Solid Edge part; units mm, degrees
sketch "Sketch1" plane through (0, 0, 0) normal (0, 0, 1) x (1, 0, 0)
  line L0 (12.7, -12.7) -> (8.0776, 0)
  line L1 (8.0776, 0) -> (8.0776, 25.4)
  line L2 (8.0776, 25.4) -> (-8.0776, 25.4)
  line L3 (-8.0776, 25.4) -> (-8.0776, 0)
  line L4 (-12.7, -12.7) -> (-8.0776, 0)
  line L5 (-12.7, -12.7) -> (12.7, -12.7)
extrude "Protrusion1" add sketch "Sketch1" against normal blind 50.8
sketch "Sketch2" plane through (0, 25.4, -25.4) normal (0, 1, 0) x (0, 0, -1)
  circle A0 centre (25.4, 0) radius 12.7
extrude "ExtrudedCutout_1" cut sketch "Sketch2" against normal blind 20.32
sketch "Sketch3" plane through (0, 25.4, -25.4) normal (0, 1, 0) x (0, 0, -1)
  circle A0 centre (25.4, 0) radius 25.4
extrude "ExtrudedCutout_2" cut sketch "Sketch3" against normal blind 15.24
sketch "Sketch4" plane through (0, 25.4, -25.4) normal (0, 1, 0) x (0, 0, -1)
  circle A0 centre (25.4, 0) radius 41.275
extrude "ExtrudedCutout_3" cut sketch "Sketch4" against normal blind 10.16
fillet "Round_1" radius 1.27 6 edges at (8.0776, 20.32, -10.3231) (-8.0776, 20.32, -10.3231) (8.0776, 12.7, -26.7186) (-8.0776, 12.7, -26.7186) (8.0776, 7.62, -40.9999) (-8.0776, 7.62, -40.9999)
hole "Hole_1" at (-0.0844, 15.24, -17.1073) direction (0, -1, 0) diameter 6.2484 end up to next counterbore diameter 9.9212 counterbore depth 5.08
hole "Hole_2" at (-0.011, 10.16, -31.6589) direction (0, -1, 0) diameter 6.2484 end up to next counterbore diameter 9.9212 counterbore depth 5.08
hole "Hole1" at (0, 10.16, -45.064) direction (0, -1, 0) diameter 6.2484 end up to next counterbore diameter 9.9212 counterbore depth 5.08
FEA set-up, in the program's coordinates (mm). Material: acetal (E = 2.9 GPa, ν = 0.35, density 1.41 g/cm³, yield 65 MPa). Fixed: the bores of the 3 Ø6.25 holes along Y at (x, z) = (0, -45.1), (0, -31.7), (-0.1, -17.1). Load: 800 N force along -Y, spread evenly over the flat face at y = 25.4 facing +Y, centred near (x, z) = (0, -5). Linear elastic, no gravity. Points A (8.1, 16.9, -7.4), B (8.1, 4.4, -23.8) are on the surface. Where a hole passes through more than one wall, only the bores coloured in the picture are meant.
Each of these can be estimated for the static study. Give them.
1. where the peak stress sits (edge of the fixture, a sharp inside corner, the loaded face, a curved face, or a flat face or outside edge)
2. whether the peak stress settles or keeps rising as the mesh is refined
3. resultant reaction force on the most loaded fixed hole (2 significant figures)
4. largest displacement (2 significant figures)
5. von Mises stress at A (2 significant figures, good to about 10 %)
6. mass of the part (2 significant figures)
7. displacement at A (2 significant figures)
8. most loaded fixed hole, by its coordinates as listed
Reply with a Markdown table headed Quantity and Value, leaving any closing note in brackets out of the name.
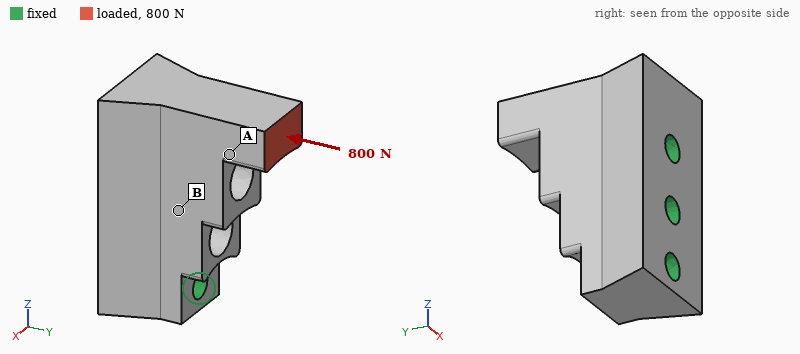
| Quantity | Value |
|---|---|
| where the peak stress sits | edge of the fixture |
| whether the peak stress settles or keeps rising as the mesh is refined | keeps rising |
| resultant reaction force on the most loaded fixed hole | 860 N |
| largest displacement | 0.11 mm |
| von Mises stress at A | 4.4 MPa |
| mass of the part | 31 g |
| displacement at A | 0.054 mm |
| most loaded fixed hole, by its coordinates as listed | (-0.1, -17.1) |
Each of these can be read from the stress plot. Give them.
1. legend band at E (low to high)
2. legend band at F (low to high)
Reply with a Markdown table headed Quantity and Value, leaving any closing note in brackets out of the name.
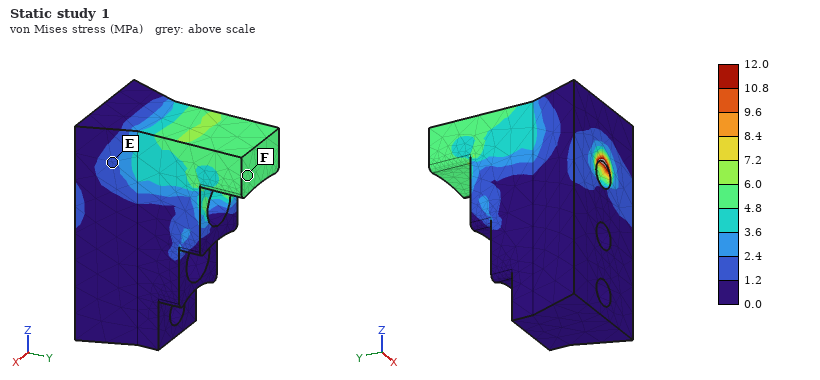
| Quantity | Value |
|---|---|
| legend band at E | 1.2 to 2.4 MPa |
| legend band at F | 4.8 to 6.0 MPa |
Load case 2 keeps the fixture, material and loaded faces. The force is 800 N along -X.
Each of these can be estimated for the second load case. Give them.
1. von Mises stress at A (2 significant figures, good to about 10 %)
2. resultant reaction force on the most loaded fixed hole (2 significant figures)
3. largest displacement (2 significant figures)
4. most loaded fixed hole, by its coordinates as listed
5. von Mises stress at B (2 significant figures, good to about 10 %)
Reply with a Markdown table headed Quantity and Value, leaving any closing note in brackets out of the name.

| Quantity | Value |
|---|---|
| von Mises stress at A | 17 MPa |
| resultant reaction force on the most loaded fixed hole | 1.0 kN |
| largest displacement | 0.52 mm |
| most loaded fixed hole, by its coordinates as listed | (-0.1, -17.1) |
| von Mises stress at B | 4.9 MPa |
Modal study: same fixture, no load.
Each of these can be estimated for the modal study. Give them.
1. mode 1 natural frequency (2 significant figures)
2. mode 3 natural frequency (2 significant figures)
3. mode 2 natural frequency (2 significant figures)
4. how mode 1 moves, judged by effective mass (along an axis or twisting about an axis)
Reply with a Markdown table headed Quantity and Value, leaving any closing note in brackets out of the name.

| Quantity | Value |
|---|---|
| mode 1 natural frequency | 4800 Hz |
| mode 3 natural frequency | 7600 Hz |
| mode 2 natural frequency | 5700 Hz |
| how mode 1 moves, judged by effective mass | along X |
